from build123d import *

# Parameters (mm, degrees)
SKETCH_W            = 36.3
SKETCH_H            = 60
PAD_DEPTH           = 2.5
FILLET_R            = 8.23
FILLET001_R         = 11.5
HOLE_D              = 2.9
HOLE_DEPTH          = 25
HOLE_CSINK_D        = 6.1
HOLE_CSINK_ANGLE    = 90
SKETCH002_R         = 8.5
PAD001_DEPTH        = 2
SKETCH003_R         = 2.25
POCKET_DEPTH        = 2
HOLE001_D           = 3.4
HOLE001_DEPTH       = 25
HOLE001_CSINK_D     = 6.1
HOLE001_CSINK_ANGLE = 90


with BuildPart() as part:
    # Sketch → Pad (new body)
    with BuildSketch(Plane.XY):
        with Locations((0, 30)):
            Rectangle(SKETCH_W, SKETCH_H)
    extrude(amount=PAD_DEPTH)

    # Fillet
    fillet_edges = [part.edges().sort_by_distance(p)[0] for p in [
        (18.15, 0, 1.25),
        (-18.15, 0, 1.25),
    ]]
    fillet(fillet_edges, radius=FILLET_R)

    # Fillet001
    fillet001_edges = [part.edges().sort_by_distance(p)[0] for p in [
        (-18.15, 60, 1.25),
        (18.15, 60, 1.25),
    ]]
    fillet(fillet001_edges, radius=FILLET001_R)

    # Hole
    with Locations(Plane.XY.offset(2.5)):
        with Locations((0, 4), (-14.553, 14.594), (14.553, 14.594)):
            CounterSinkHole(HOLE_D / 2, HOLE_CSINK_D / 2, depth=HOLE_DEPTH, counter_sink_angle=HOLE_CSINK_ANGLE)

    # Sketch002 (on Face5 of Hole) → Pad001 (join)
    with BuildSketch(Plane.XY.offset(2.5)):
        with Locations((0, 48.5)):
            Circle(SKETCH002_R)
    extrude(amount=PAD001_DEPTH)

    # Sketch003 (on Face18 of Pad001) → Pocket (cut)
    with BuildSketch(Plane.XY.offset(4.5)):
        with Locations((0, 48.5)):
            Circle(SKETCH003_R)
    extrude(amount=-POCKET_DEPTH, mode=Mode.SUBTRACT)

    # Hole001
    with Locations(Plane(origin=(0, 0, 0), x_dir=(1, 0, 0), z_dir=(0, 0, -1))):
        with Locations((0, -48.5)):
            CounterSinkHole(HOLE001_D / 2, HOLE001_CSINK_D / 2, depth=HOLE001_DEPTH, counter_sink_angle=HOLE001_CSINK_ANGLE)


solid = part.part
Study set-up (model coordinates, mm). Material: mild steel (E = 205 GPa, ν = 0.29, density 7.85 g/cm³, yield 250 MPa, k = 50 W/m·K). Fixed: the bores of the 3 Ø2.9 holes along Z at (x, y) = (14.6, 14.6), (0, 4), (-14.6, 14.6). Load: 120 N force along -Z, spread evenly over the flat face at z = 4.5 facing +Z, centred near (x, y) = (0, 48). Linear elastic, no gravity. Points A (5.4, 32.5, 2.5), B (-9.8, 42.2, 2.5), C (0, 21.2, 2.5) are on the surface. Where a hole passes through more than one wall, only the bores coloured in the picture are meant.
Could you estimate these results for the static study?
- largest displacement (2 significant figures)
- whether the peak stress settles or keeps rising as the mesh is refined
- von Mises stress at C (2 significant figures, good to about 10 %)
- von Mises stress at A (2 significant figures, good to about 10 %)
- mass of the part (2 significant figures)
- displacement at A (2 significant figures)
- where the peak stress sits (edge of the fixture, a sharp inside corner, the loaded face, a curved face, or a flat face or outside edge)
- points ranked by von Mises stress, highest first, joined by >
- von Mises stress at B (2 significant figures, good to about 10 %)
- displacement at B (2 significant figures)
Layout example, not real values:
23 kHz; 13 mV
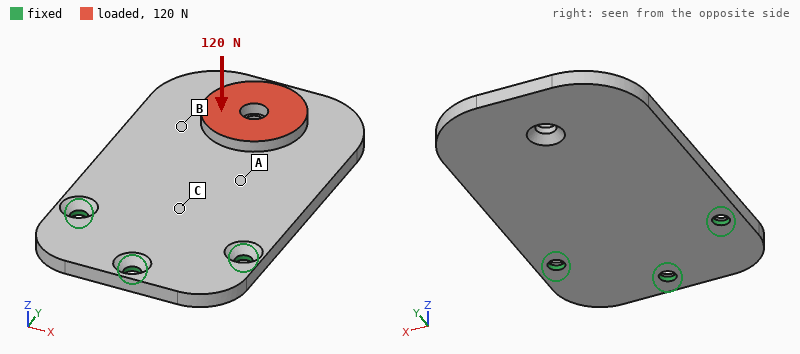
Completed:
0.32 mm; keeps rising; 90 MPa; 53 MPa; 43 g; 0.092 mm; edge of the fixture; C > A > B; 20 MPa; 0.17 mm
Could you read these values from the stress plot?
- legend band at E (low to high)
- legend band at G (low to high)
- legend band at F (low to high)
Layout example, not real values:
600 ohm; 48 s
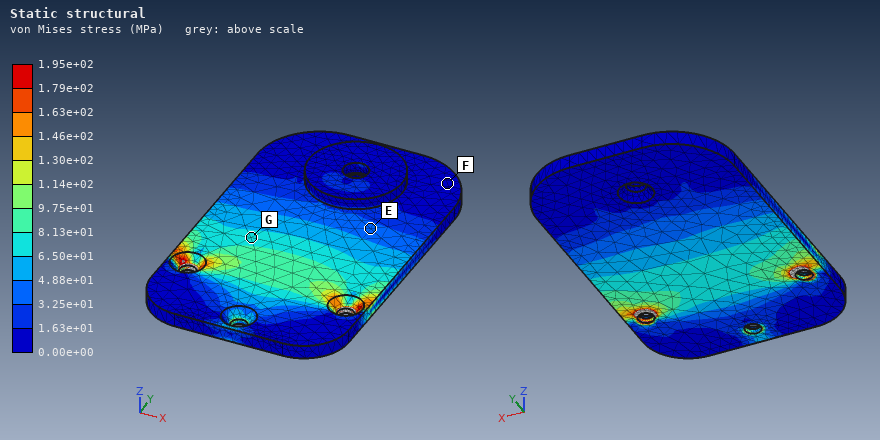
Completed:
3.25e+01 to 4.88e+01 MPa; 6.50e+01 to 8.13e+01 MPa; 0.00e+00 to 1.63e+01 MPa
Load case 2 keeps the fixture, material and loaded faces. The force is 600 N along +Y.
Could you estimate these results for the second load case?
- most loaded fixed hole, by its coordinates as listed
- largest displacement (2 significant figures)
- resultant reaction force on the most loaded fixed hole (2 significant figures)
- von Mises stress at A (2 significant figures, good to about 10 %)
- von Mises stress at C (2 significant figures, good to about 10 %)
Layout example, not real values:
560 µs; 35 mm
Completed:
(0, 4); 0.23 mm; 320 N; 58 MPa; 58 MPa
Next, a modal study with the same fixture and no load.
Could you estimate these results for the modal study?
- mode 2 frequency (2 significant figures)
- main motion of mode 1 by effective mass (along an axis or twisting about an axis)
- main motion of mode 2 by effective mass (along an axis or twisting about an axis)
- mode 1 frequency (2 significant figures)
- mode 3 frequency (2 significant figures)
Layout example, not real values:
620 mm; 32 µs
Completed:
3200 Hz; along Z; twisting about Y; 830 Hz; 5600 Hz
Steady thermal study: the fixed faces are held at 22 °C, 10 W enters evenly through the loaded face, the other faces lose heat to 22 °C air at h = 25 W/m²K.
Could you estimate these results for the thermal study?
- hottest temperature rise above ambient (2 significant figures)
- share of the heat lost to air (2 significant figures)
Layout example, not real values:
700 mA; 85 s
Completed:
66 K; 34 %
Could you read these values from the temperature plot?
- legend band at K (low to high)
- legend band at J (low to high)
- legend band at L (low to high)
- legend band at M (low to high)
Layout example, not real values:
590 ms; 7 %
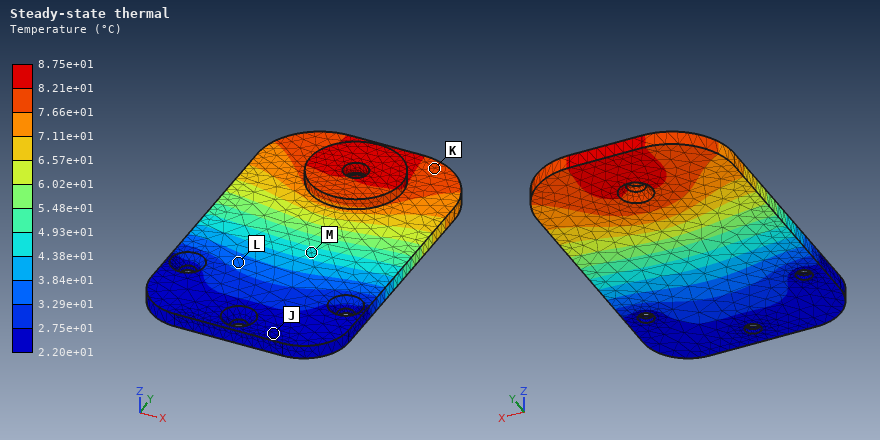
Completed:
7.66e+01 to 8.21e+01 °C; 2.20e+01 to 2.75e+01 °C; 3.29e+01 to 3.84e+01 °C; 4.38e+01 to 4.93e+01 °C
